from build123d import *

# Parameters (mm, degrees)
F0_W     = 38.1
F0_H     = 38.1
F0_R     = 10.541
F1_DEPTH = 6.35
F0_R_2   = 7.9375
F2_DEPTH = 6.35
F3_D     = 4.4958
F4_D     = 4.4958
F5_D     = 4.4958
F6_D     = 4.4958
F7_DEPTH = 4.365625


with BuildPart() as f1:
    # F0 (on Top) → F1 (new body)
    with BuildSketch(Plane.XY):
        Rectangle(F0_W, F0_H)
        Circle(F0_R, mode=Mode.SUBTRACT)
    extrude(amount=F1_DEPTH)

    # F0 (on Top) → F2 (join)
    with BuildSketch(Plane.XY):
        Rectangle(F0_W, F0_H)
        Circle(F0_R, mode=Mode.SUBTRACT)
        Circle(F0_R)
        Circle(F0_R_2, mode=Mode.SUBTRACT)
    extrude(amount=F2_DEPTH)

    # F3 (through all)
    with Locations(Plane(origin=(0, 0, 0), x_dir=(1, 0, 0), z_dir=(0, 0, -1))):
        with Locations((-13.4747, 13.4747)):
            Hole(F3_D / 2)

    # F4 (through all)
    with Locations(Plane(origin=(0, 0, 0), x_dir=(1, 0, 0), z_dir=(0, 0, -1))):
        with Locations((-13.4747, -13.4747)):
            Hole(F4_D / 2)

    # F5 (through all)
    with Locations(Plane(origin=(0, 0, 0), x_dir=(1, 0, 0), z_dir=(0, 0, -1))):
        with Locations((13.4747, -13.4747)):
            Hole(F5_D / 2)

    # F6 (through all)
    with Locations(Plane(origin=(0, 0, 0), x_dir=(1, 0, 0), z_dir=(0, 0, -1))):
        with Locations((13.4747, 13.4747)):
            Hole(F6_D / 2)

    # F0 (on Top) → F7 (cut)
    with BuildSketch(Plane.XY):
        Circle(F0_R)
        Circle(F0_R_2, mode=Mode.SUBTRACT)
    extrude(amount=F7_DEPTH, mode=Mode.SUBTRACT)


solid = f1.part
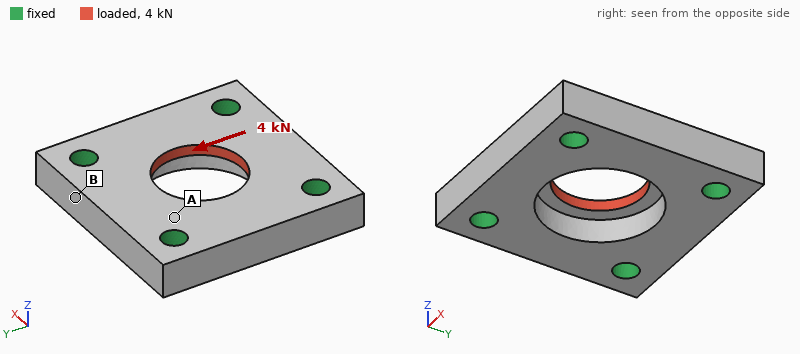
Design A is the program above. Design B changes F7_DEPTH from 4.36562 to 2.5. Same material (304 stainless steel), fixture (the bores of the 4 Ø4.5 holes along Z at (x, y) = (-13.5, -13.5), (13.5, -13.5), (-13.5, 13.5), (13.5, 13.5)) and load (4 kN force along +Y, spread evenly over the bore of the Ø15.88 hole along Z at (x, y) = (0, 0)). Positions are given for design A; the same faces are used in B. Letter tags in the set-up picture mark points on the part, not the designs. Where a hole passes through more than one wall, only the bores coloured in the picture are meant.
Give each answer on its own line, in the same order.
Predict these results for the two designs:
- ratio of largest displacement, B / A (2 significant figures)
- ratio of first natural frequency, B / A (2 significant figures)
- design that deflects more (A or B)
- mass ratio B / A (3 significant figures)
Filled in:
0.63
0.95
A
1.04
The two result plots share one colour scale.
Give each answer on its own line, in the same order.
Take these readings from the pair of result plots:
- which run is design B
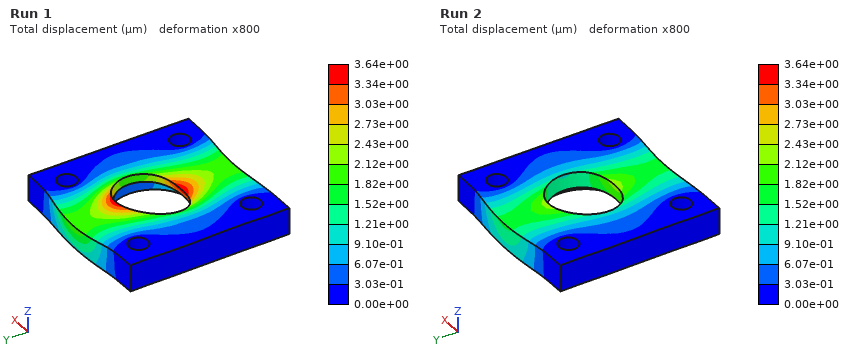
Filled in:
Run 2
